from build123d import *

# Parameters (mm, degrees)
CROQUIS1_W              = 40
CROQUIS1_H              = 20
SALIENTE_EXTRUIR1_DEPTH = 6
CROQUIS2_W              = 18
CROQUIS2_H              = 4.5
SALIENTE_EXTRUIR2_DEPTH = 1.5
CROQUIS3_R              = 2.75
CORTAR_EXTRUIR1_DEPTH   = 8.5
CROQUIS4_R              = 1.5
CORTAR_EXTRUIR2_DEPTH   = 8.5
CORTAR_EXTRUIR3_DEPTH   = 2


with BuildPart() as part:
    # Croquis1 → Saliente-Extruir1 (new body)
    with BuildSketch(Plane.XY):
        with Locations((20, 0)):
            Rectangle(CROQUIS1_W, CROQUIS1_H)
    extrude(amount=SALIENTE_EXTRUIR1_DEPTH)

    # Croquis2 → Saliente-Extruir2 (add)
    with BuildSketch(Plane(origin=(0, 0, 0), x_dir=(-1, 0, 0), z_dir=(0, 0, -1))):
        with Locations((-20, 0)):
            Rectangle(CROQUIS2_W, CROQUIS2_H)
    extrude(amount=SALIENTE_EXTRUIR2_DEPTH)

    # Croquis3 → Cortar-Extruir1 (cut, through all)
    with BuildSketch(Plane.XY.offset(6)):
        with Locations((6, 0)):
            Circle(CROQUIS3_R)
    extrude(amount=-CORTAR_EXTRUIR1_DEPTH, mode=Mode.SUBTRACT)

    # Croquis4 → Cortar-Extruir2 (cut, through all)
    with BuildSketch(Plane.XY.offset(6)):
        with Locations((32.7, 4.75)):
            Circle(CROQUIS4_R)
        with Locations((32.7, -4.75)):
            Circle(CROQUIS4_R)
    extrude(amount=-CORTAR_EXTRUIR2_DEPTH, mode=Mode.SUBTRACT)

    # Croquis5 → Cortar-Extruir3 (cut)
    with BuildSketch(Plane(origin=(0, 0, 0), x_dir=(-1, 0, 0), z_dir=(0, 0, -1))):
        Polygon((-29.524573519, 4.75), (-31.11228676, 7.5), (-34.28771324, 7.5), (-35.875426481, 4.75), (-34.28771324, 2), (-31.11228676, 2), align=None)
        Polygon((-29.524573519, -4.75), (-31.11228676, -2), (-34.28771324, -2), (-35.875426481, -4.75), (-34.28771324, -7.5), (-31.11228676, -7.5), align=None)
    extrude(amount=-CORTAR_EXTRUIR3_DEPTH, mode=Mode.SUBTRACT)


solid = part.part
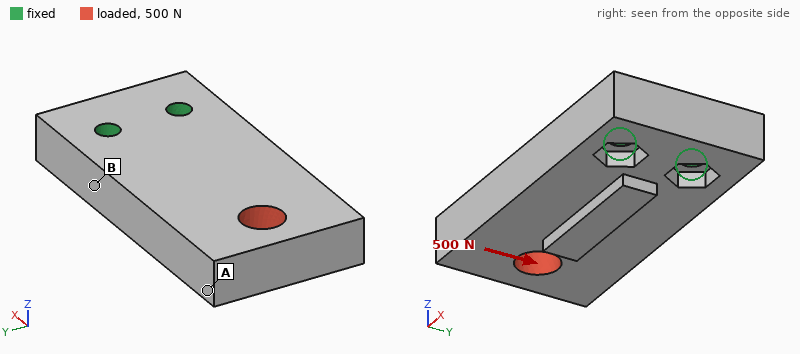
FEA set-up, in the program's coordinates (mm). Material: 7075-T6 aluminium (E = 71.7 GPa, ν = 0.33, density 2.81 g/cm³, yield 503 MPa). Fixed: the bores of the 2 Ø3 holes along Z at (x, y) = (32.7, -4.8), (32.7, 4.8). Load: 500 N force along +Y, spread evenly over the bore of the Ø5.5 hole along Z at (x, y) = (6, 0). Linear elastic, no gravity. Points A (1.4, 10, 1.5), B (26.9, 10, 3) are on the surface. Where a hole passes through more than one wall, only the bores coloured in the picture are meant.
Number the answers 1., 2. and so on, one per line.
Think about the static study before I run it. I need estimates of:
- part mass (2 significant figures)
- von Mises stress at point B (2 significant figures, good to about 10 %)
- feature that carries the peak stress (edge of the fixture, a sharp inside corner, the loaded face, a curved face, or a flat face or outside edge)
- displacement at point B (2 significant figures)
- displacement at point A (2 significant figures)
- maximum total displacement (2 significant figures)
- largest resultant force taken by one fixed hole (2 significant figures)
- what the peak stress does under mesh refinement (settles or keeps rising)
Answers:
1. 13 g
2. 23 MPa
3. edge of the fixture
4. 6.2 µm
5. 28 µm
6. 30 µm
7. 1.2 kN
8. keeps rising
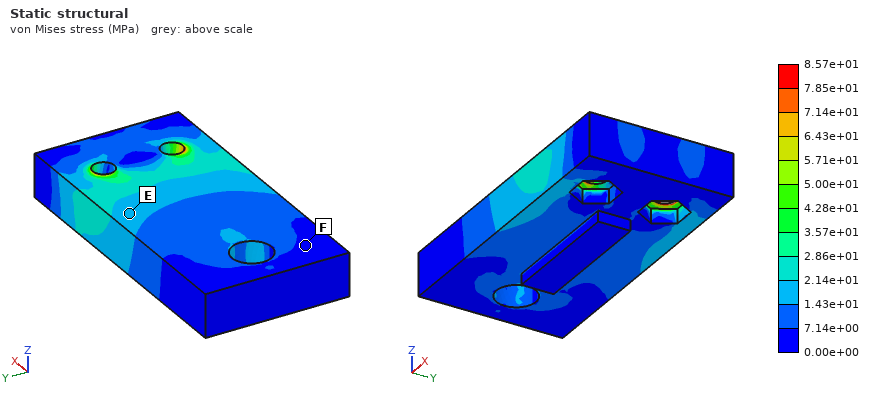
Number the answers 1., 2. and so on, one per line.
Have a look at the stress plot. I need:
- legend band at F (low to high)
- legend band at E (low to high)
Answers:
1. 0.00e+00 to 7.14e+00 MPa
2. 1.43e+01 to 2.14e+01 MPa
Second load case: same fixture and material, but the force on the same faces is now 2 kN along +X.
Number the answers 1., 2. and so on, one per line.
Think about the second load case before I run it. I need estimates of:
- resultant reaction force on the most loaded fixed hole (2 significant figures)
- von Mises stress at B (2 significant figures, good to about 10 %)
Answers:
1. 1.0 kN
2. 14 MPa
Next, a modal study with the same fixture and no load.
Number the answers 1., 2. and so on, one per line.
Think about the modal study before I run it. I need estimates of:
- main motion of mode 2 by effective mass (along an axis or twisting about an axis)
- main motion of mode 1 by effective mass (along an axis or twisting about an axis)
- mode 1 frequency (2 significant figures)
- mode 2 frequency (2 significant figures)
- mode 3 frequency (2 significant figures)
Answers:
1. along Y
2. along Z
3. 4000 Hz
4. 10 kHz
5. 13 kHz
